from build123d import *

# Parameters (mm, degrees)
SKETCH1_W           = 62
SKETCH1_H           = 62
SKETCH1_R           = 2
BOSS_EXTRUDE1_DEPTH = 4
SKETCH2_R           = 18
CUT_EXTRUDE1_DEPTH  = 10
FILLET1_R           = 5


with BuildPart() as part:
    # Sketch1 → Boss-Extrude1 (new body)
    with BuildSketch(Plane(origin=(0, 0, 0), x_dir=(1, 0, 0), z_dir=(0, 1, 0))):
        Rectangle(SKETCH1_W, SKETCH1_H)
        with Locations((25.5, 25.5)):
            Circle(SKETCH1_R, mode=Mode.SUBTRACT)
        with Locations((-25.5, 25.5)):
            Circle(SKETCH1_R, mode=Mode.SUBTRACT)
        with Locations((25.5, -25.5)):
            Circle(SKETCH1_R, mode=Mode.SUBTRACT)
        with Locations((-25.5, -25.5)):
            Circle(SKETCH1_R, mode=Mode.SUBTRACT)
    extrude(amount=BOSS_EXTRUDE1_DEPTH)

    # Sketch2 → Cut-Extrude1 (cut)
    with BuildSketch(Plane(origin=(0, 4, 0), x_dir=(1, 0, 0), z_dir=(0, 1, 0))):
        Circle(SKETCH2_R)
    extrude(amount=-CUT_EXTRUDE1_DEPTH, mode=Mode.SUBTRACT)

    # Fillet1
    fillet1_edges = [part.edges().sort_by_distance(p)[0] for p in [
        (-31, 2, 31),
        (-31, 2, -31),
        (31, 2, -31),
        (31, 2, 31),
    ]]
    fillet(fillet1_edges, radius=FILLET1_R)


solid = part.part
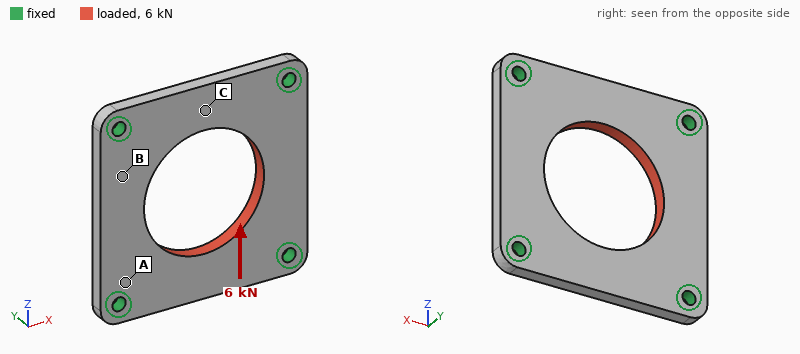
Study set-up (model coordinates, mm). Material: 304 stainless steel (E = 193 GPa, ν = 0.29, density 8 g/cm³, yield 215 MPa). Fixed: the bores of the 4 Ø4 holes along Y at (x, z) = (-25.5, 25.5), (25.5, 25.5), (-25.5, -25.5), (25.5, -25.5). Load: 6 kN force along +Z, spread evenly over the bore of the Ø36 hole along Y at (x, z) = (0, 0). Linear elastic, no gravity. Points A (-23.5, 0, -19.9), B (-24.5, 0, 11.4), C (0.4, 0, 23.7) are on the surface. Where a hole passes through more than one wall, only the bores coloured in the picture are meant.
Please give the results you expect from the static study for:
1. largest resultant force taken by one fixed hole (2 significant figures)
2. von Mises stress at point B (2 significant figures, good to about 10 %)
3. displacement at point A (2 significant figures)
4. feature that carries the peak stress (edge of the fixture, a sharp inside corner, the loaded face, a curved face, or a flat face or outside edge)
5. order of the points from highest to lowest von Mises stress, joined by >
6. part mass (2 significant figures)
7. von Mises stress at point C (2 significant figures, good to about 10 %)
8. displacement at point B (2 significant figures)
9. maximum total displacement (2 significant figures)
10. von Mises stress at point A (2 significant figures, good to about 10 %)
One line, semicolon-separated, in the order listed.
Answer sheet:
1.6 kN; 19 MPa; 1.2 µm; edge of the fixture; A > B > C; 88 g; 8.9 MPa; 2.0 µm; 6.8 µm; 31 MPa
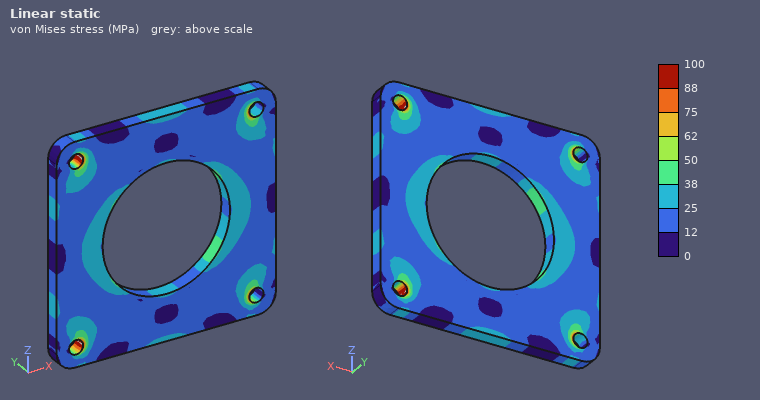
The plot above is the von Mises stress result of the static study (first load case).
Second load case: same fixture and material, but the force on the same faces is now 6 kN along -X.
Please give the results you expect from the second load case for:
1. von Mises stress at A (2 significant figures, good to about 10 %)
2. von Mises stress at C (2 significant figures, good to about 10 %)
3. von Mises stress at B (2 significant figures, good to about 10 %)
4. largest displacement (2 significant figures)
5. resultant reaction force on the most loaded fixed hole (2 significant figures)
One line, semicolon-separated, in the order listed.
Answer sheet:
25 MPa; 26 MPa; 19 MPa; 6.8 µm; 1.6 kN
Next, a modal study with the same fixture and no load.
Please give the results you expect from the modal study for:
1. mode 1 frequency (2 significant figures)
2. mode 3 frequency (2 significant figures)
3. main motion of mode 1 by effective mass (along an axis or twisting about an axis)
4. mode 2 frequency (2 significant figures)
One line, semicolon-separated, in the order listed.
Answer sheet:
7000 Hz; 8200 Hz; along Y; 8200 Hz
